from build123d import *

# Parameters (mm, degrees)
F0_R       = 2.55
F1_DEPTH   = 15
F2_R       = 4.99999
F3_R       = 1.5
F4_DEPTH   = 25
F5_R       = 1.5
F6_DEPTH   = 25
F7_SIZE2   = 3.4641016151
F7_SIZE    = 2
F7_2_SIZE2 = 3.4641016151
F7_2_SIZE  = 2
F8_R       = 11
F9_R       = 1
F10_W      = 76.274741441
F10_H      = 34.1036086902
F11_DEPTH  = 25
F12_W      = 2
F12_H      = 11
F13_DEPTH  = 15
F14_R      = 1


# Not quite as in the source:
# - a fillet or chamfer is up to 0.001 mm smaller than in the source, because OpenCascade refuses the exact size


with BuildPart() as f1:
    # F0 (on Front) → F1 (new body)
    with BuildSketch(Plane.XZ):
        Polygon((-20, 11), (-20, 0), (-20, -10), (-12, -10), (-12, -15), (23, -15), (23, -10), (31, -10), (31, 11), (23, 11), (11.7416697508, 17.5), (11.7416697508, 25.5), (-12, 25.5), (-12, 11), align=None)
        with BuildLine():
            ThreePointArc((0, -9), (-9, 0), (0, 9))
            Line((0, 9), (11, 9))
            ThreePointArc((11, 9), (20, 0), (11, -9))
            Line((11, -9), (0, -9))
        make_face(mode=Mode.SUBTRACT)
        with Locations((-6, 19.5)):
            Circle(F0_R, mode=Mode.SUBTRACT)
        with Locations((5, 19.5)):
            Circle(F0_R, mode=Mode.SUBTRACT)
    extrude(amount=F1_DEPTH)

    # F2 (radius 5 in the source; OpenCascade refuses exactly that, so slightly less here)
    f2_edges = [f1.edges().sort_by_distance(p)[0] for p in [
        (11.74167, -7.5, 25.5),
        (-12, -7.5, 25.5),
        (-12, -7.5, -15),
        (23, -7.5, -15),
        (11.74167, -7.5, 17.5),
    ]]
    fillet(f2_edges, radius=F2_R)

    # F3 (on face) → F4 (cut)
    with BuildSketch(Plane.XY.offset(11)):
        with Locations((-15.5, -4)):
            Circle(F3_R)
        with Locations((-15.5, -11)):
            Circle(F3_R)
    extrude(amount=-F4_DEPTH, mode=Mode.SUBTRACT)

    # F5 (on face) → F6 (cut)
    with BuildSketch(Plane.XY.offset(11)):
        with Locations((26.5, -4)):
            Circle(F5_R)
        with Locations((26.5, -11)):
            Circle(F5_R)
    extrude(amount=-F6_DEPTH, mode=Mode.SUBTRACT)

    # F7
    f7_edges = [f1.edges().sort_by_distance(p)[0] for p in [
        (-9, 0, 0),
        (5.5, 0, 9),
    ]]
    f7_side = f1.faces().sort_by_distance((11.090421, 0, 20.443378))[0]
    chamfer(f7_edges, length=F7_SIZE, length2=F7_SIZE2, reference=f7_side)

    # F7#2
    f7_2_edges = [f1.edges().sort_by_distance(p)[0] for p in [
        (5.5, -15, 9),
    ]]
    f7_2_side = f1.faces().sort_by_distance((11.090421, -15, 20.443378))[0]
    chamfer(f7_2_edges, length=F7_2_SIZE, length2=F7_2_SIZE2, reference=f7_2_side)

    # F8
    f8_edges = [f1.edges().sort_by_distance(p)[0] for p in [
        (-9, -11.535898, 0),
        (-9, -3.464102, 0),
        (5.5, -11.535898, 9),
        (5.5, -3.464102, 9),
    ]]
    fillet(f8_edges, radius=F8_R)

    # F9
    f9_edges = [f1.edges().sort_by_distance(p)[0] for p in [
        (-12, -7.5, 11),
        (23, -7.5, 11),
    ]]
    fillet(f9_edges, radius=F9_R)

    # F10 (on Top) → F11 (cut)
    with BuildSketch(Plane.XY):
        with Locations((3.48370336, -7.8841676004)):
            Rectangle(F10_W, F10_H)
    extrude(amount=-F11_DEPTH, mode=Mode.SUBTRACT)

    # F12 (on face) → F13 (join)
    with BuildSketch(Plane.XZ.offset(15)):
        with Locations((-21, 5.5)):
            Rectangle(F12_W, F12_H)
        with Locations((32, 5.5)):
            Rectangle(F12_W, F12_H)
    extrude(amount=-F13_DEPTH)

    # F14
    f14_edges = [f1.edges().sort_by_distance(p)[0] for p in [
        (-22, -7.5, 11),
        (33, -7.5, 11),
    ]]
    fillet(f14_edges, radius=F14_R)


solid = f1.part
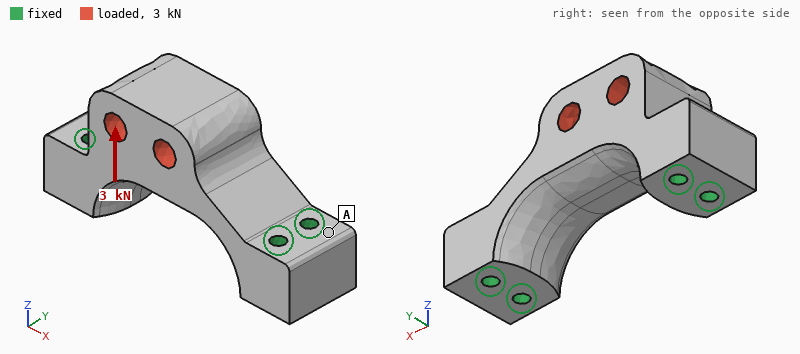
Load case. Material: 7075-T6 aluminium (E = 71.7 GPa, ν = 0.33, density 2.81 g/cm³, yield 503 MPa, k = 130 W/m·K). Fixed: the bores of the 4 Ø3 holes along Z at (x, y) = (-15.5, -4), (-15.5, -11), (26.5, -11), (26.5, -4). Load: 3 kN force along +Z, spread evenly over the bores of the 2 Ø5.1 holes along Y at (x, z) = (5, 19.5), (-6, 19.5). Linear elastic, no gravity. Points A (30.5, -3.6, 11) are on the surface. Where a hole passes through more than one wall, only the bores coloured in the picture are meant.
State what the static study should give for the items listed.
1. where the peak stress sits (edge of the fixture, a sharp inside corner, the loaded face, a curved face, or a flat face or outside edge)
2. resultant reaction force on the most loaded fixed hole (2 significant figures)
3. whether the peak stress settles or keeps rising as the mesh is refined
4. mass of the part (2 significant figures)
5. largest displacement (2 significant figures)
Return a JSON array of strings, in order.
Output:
["edge of the fixture", "1.2 kN", "keeps rising", "28 g", "8.8 µm"]
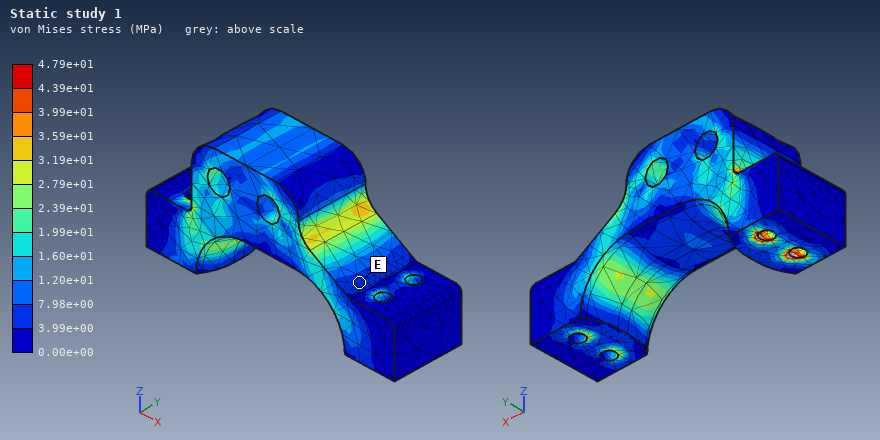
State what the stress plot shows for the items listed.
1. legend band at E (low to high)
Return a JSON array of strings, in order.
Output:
["3.99e+00 to 7.98e+00 MPa"]
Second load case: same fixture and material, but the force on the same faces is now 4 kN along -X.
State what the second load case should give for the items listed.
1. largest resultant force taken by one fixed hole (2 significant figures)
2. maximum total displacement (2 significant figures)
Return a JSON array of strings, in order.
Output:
["1.2 kN", "12 µm"]
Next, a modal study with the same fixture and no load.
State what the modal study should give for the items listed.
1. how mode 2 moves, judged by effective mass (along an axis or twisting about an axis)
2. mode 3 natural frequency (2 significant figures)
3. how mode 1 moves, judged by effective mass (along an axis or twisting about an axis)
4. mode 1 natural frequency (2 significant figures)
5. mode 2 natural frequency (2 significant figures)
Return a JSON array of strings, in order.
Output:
["along Z", "30 kHz", "along Y", "13 kHz", "24 kHz"]
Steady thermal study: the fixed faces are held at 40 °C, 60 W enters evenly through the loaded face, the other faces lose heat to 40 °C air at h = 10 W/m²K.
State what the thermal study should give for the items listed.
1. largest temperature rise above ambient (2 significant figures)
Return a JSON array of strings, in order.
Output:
["37 K"]
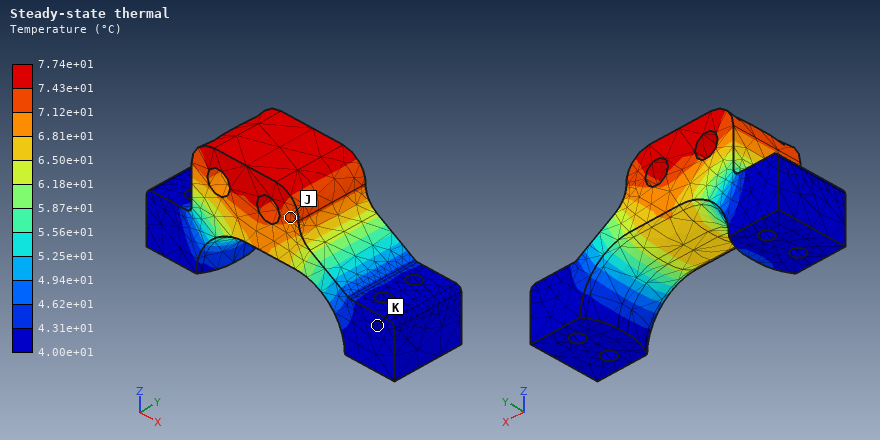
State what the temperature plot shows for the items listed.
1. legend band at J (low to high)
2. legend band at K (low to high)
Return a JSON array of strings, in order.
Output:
["7.12e+01 to 7.43e+01 °C", "4.00e+01 to 4.31e+01 °C"]
